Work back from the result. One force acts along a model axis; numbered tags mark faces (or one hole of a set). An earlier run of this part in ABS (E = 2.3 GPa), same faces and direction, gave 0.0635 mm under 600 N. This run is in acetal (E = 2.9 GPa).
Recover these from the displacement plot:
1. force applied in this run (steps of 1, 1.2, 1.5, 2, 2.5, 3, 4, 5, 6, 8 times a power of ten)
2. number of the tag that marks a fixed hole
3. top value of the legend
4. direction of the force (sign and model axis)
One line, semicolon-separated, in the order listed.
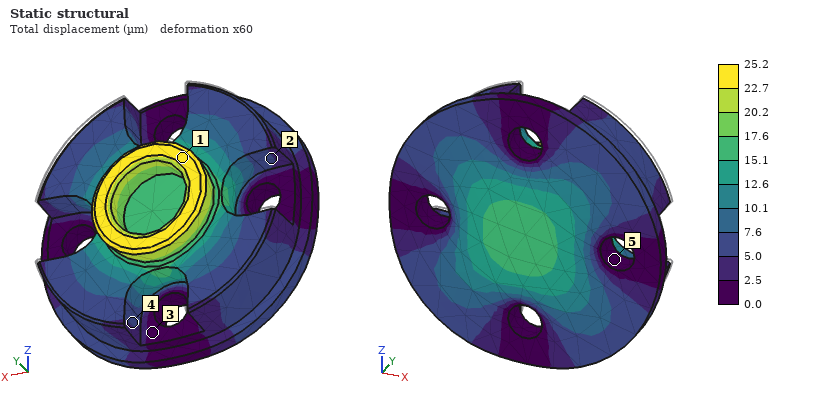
300 N; 5; 25.2 µm; -Y
